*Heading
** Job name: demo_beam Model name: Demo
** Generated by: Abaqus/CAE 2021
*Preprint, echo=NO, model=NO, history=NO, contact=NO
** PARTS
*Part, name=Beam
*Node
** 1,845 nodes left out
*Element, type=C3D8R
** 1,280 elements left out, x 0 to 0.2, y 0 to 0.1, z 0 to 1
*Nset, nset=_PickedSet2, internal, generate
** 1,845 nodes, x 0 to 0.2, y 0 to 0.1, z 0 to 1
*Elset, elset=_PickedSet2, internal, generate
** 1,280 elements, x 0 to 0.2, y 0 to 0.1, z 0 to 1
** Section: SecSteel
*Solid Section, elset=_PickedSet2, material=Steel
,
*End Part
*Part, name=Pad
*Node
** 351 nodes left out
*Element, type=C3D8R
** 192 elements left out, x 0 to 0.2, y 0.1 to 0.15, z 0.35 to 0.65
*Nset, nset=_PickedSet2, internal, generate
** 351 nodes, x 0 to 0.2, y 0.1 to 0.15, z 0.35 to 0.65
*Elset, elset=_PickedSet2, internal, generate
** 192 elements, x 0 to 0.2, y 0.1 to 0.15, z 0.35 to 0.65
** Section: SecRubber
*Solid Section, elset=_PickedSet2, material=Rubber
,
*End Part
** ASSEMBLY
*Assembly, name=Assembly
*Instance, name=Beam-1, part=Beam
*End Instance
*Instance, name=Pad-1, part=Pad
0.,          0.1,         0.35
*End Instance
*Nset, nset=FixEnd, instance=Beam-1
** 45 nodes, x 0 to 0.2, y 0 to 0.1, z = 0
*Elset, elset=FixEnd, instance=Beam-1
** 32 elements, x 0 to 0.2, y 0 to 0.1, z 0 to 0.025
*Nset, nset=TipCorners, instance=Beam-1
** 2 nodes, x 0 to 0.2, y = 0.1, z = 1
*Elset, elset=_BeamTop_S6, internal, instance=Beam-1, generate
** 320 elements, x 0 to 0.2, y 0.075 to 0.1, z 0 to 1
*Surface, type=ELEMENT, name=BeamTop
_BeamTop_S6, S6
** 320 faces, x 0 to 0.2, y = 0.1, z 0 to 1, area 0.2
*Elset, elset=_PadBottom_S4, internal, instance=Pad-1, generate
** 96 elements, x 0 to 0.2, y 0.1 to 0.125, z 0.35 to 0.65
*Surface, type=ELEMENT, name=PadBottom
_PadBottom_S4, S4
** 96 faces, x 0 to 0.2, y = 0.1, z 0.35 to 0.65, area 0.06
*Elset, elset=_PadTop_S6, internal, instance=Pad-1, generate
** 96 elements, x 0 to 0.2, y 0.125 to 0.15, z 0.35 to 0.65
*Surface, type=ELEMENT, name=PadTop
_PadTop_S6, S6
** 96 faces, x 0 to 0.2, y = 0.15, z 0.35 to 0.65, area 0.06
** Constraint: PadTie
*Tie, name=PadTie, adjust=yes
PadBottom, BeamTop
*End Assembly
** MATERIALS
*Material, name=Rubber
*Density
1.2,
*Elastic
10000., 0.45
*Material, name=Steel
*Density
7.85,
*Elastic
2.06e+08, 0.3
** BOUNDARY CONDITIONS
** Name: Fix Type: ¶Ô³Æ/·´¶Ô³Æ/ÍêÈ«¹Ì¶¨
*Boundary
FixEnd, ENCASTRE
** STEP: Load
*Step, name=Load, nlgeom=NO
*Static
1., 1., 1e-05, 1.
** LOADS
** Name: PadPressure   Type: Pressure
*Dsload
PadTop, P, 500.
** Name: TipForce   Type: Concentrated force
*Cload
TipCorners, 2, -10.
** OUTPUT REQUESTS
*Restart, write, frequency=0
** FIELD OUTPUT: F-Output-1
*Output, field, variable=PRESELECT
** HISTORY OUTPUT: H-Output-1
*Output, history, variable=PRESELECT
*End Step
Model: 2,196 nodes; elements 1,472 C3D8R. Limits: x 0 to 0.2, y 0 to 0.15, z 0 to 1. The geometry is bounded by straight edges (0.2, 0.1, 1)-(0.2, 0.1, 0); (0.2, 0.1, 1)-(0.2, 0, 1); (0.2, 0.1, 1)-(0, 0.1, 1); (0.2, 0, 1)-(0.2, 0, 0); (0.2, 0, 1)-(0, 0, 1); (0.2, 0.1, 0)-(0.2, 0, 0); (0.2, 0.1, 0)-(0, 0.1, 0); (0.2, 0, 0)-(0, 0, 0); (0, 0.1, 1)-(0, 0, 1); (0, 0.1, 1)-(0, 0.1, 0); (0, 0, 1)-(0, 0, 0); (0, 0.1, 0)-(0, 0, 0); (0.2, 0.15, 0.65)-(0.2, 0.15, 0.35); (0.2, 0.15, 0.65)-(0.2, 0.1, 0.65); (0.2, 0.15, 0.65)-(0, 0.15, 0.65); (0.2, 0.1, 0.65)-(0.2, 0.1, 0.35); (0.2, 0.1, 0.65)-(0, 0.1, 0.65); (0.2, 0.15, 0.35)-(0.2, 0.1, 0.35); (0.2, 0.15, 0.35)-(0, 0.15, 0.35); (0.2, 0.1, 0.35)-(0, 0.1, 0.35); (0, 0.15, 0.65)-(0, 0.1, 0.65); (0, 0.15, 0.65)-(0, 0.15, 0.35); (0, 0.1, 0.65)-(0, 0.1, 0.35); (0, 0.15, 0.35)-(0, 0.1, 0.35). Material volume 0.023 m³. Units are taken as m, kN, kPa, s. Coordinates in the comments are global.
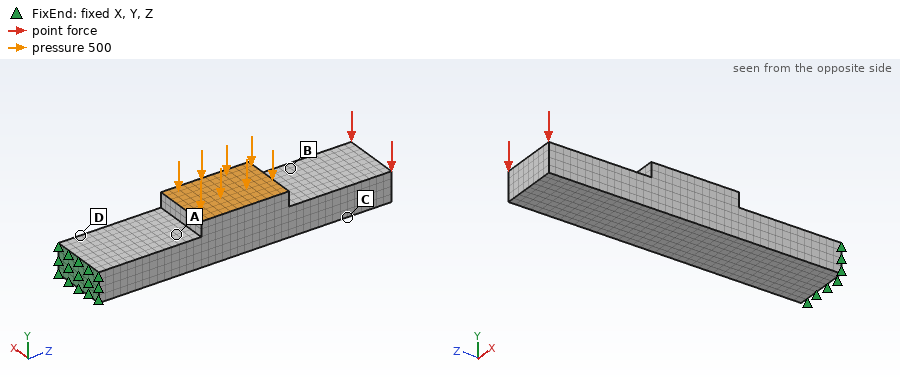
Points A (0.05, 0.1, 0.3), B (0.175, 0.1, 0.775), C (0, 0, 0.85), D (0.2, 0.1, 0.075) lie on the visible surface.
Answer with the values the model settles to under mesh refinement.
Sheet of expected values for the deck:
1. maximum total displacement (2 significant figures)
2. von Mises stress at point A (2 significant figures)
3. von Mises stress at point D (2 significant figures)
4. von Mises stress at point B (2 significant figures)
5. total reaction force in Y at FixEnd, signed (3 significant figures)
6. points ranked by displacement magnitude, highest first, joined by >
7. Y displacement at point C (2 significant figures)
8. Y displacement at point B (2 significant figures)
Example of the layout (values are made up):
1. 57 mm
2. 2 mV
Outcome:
1. 0.0054 m
2. 60000 kPa
3. 91000 kPa
4. 14000 kPa
5. 50.0 kN
6. C > B > A > D
7. -0.0023 m
8. -0.0020 m
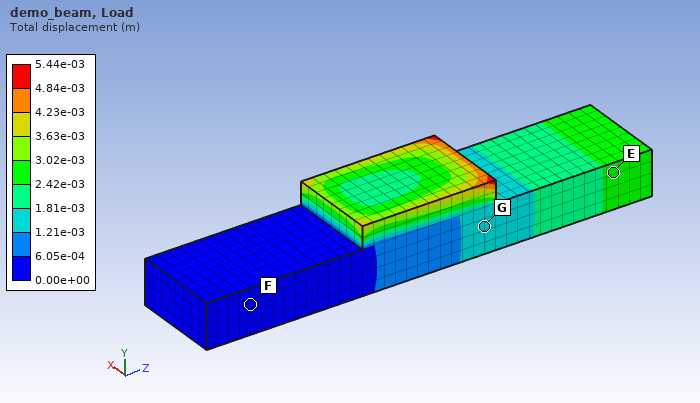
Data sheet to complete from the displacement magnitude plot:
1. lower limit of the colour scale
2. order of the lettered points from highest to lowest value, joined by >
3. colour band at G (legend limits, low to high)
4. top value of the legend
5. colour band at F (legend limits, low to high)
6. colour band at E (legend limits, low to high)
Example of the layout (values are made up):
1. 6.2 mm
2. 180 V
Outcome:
1. 0.00e+00 m
2. E > G > F
3. 1.21e-03 to 1.81e-03 m
4. 5.44e-03 m
5. 0.00e+00 to 6.05e-04 m
6. 2.42e-03 to 3.02e-03 m
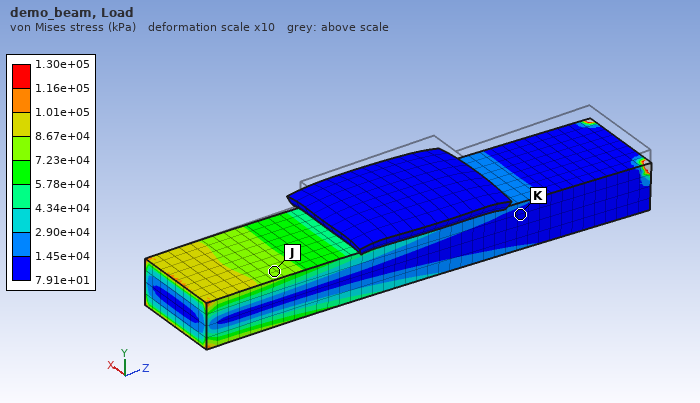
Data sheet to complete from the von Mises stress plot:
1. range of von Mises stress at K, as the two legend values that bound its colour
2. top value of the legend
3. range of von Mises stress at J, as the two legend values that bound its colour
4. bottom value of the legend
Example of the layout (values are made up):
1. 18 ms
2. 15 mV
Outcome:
1. 7.91e+01 to 1.45e+04 kPa
2. 1.30e+05 kPa
3. 7.23e+04 to 8.67e+04 kPa
4. 7.91e+01 kPa
